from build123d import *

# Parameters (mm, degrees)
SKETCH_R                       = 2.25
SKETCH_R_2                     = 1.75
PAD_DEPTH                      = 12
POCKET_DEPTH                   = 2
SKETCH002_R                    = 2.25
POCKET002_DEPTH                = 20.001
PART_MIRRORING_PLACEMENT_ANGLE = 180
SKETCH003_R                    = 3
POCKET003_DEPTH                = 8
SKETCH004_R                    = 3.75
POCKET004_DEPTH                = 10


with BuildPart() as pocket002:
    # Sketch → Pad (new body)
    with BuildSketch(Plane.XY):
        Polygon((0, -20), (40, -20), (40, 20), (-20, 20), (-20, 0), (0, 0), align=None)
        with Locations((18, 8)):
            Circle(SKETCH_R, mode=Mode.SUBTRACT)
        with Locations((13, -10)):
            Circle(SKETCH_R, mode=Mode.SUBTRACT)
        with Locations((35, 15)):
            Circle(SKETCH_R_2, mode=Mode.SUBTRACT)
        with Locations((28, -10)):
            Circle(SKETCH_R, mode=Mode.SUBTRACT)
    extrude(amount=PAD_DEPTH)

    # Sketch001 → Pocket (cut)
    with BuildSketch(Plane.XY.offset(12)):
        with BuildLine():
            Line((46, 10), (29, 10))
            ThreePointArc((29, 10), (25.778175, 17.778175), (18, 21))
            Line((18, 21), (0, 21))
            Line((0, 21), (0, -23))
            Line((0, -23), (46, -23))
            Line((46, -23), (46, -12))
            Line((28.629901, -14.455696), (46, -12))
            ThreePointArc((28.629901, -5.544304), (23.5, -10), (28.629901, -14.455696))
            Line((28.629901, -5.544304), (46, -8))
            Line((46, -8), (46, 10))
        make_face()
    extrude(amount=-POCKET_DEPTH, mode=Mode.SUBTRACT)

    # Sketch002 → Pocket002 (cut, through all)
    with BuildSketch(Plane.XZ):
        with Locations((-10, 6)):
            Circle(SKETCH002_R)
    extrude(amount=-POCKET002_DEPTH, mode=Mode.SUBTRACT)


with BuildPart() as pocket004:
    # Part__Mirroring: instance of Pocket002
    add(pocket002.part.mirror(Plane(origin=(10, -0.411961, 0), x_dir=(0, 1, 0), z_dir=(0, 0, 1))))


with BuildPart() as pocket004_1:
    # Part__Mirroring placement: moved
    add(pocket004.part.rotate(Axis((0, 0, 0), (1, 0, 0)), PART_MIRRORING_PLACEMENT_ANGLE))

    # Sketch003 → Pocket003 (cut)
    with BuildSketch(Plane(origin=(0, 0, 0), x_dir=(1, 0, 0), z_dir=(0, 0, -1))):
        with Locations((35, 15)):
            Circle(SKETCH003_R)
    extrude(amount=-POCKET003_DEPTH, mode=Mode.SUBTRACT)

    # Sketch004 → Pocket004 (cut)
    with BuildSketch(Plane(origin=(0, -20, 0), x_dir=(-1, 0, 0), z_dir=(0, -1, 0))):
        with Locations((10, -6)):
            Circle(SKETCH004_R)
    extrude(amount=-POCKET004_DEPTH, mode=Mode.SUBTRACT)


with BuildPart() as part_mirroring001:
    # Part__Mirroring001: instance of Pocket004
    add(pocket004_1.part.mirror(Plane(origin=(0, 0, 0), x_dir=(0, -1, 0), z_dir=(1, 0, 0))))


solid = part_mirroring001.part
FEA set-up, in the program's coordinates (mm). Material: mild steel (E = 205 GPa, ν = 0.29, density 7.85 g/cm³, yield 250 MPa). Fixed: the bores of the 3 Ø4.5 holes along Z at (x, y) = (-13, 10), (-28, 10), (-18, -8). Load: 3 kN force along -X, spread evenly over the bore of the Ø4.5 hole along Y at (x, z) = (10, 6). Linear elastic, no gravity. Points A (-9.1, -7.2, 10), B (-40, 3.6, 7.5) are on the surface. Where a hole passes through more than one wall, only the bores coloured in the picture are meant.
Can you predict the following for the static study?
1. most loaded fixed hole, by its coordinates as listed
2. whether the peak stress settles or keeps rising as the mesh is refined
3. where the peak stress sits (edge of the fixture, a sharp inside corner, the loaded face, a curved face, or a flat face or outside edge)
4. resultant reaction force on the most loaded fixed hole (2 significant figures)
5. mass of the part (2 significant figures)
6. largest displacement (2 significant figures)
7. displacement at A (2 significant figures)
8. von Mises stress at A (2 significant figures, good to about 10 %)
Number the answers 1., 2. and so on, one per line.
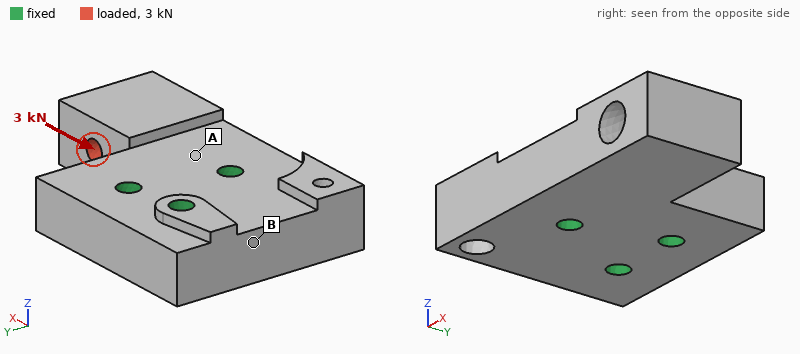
1. (-18, -8)
2. keeps rising
3. a sharp inside corner
4. 2.3 kN
5. 160 g
6. 6.1 µm
7. 1.0 µm
8. 26 MPa
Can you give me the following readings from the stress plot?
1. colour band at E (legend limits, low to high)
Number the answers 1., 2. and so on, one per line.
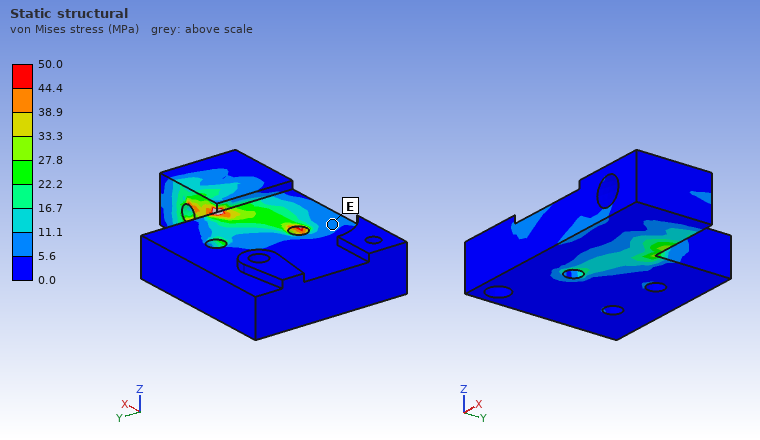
1. 5.6 to 11.1 MPa
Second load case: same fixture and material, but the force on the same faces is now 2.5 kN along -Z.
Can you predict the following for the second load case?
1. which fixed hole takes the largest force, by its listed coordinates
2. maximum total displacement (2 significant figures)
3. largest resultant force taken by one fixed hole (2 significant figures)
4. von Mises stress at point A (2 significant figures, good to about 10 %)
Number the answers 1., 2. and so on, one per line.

1. (-13, 10)
2. 63 µm
3. 1.8 kN
4. 100 MPa
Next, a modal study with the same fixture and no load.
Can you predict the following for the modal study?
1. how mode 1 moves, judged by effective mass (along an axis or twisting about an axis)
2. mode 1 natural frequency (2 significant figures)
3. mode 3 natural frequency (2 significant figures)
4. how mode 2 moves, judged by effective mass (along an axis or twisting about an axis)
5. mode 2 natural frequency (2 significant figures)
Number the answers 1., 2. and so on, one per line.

1. along Z
2. 6200 Hz
3. 18 kHz
4. along Y
5. 13 kHz
